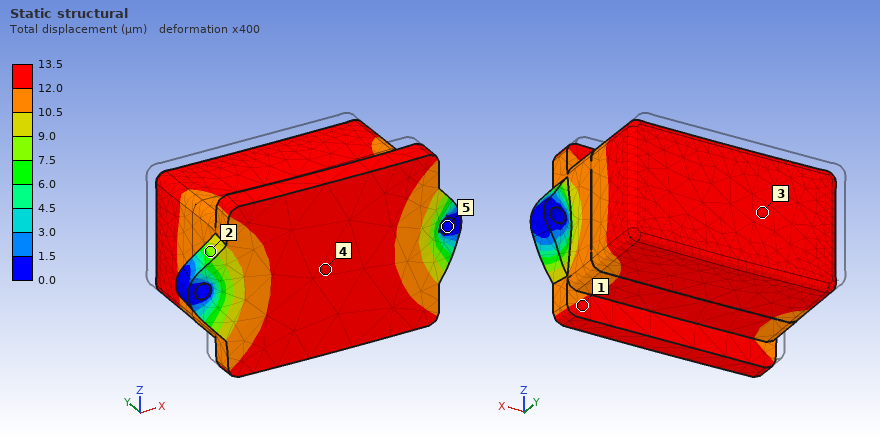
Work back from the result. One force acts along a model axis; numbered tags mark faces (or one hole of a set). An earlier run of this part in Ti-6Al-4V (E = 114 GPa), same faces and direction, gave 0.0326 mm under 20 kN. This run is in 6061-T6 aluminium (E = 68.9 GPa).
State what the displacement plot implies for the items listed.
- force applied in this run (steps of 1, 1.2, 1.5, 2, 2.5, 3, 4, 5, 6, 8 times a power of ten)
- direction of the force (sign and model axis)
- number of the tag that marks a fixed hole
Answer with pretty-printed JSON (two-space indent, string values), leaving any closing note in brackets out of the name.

{
  "force applied in this run": "5 kN",
  "direction of the force": "-Y",
  "number of the tag that marks a fixed hole": "5"
}
